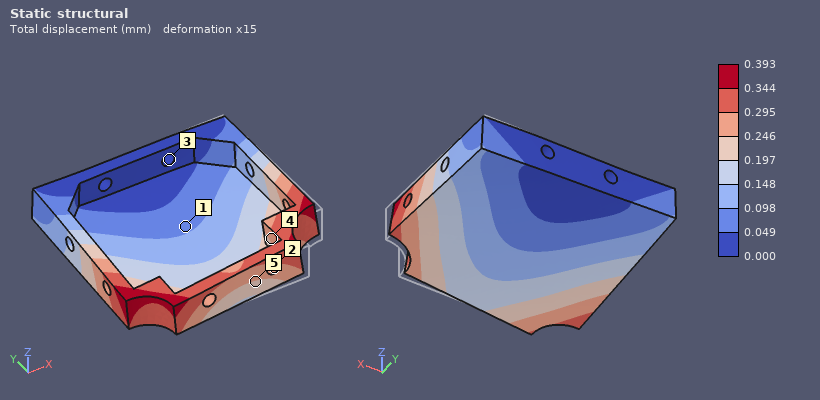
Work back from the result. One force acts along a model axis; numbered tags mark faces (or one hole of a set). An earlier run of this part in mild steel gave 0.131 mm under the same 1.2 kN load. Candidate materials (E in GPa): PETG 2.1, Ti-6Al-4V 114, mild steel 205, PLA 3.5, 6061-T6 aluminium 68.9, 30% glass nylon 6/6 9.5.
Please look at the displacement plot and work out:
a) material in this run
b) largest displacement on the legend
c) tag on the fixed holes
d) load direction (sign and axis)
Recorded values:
6061-T6 aluminium
0.393 mm
3
-X
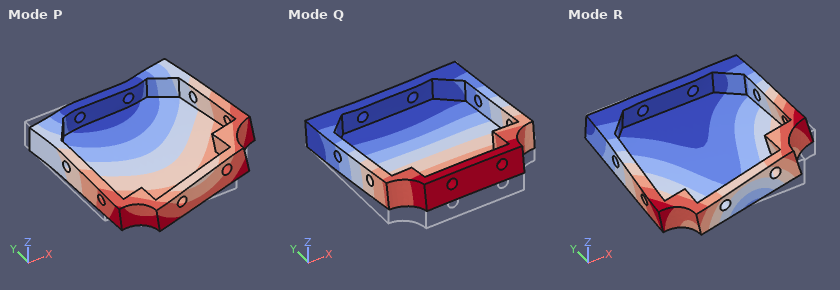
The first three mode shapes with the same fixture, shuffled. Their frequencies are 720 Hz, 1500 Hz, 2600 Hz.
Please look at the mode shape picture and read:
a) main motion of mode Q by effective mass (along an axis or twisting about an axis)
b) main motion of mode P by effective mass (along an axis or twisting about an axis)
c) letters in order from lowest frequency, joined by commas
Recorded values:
along Z
along X
Q, R, P
